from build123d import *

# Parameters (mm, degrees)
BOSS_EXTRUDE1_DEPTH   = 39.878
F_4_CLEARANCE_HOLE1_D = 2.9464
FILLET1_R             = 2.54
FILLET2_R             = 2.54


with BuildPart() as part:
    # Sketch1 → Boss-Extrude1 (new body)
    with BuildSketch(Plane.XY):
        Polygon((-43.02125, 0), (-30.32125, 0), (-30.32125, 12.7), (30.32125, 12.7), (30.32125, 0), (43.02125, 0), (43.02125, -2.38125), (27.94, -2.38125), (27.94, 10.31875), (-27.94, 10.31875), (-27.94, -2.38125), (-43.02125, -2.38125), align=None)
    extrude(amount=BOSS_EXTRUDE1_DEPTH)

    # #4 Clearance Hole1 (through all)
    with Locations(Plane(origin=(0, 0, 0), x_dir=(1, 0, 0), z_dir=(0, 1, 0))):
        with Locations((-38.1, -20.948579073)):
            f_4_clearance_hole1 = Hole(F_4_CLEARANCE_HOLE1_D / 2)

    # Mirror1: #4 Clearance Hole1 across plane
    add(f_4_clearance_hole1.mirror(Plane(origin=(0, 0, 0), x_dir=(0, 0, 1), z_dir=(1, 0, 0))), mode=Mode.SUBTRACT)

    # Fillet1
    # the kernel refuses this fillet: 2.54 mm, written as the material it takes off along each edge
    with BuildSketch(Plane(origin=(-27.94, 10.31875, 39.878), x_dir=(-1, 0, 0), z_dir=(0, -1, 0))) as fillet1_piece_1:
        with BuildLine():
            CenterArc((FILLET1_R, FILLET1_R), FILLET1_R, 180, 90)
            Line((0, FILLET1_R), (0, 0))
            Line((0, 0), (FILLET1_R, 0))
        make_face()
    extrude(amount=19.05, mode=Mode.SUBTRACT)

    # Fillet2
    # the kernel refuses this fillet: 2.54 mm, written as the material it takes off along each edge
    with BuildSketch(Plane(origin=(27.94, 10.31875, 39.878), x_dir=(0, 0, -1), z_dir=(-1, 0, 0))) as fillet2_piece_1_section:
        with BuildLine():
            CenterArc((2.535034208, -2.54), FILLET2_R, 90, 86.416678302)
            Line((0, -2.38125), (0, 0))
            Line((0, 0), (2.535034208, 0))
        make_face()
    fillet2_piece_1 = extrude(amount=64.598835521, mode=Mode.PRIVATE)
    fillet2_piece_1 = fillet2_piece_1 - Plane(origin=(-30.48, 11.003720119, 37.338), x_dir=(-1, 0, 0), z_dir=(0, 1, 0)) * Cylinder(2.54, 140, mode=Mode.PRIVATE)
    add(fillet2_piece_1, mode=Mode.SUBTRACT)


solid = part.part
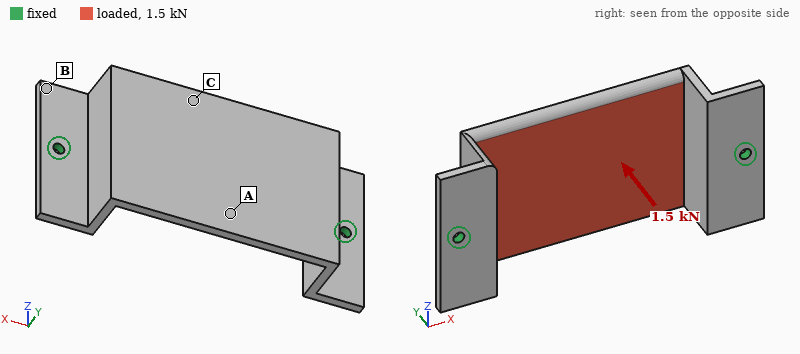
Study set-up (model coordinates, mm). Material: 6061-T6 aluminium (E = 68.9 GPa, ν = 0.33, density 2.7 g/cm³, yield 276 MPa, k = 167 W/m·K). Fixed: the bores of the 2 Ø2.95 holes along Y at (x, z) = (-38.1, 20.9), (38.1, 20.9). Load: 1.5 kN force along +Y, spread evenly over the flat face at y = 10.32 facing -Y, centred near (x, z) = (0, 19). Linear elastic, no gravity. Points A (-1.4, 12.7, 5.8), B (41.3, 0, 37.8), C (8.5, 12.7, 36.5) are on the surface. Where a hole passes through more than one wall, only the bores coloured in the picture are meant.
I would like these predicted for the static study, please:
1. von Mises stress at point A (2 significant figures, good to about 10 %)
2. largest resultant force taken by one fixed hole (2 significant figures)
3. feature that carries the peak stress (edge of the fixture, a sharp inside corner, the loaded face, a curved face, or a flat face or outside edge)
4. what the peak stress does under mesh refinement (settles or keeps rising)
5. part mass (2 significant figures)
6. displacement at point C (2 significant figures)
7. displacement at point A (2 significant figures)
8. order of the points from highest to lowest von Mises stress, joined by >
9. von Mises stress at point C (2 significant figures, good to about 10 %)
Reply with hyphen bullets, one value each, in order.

- 130 MPa
- 1.1 kN
- edge of the fixture
- keeps rising
- 28 g
- 0.25 mm
- 0.47 mm
- A > C > B
- 90 MPa
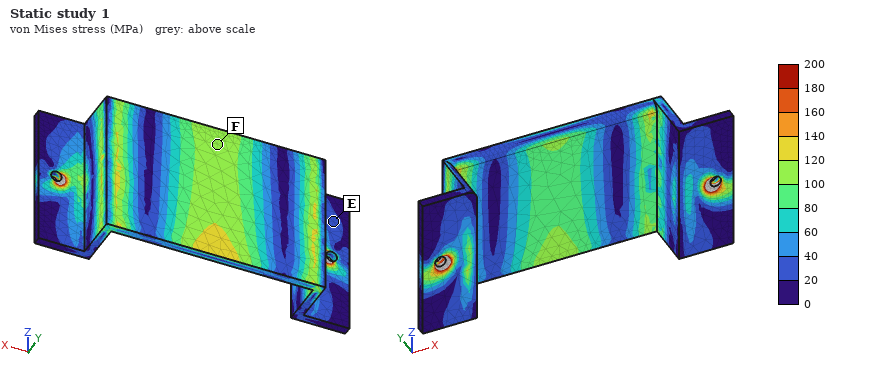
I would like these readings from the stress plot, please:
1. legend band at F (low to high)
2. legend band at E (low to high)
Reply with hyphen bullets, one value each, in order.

- 100 to 120 MPa
- 20 to 40 MPa
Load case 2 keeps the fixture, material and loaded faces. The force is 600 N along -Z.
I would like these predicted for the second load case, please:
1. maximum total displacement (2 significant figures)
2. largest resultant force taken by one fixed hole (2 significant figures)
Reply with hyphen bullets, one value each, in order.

- 0.26 mm
- 300 N
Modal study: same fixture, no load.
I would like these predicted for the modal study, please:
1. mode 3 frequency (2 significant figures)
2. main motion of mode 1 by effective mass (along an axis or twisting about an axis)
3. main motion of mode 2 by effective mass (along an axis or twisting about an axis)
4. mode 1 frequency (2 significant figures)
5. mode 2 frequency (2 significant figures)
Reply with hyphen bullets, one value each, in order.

- 3000 Hz
- along Z
- along X
- 1600 Hz
- 2800 Hz
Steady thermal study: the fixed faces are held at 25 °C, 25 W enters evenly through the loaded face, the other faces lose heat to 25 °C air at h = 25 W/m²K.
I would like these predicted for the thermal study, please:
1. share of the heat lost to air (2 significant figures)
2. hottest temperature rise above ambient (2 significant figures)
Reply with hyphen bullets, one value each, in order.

- 14 %
- 32 K
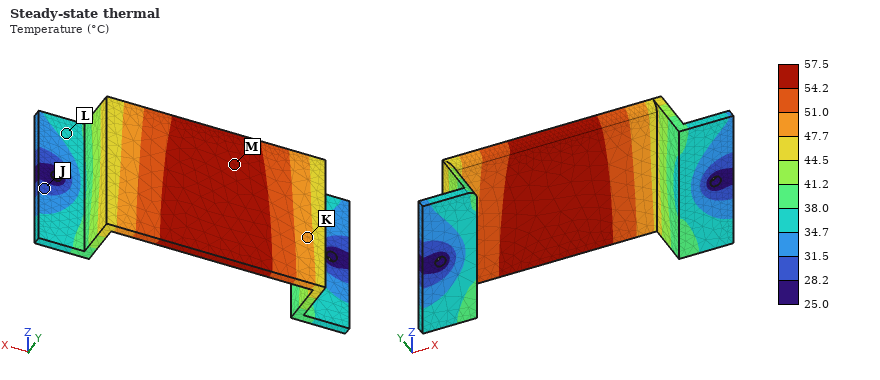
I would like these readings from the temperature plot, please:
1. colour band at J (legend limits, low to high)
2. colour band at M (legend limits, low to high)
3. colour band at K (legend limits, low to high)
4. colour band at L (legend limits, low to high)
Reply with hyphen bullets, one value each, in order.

- 28.2 to 31.5 °C
- 54.2 to 57.5 °C
- 47.7 to 51.0 °C
- 34.7 to 38.0 °C
